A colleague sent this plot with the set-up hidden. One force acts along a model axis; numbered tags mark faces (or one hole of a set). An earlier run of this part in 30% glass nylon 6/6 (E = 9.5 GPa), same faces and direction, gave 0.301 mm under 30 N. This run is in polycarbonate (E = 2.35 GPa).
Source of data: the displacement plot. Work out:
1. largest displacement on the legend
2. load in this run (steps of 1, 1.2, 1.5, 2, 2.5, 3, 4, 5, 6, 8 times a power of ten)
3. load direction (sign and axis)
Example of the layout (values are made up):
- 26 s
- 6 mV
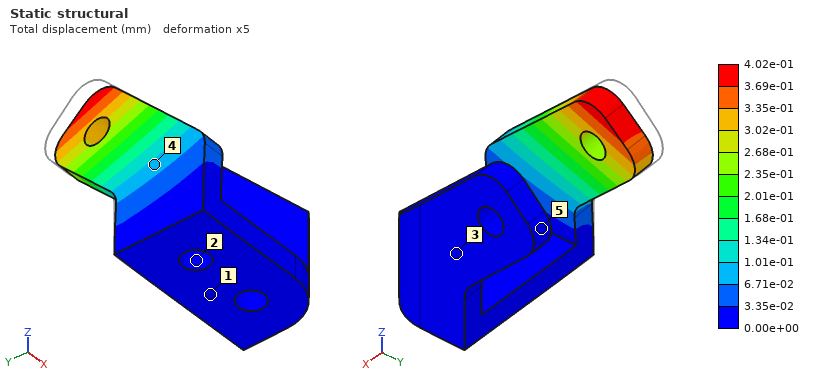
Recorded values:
- 4.02e-01 mm
- 10 N
- +X
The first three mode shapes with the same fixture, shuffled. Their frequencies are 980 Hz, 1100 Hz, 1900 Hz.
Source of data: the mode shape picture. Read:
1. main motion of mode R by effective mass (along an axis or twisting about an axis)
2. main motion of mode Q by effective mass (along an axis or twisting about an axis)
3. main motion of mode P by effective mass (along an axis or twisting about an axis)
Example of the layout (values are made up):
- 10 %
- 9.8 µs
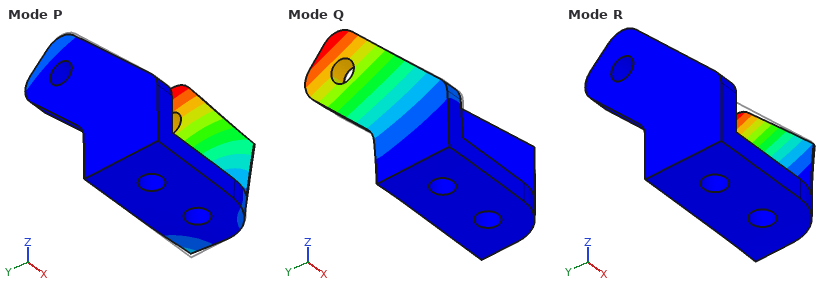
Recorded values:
- along X
- along X
- along Y
